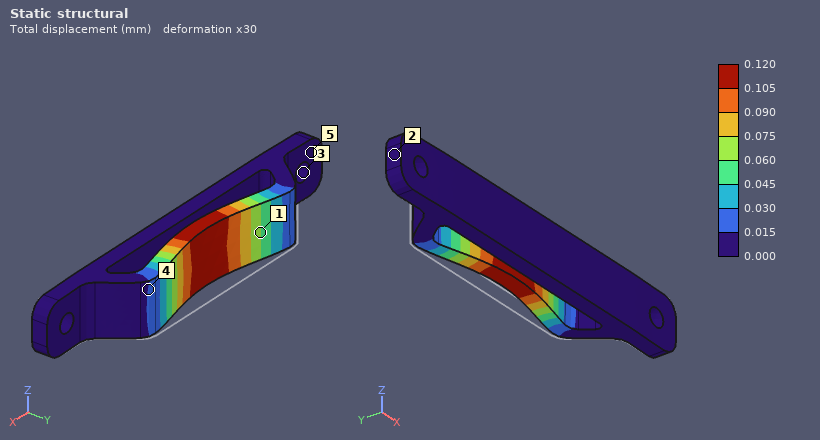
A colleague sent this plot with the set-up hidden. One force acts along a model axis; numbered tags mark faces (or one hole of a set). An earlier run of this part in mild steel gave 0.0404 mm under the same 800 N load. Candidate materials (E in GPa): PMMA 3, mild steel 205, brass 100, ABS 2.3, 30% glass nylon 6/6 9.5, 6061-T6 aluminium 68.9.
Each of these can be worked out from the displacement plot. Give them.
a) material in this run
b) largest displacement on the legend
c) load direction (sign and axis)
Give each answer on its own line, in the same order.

6061-T6 aluminium
0.120 mm
-Y
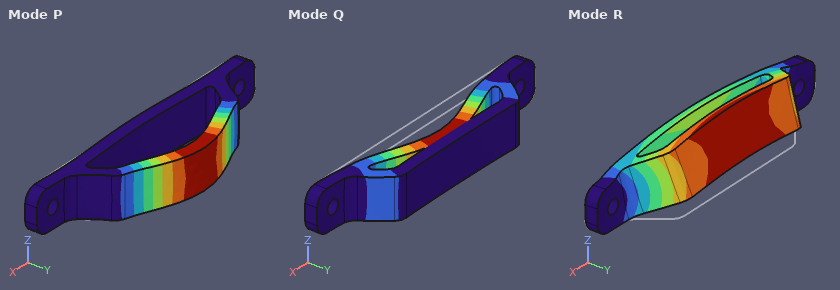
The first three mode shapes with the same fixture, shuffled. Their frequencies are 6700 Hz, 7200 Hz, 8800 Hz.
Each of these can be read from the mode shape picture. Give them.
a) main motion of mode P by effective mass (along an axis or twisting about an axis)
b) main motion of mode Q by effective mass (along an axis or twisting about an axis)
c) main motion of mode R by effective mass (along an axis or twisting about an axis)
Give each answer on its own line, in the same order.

along Y
along Y
along Z
